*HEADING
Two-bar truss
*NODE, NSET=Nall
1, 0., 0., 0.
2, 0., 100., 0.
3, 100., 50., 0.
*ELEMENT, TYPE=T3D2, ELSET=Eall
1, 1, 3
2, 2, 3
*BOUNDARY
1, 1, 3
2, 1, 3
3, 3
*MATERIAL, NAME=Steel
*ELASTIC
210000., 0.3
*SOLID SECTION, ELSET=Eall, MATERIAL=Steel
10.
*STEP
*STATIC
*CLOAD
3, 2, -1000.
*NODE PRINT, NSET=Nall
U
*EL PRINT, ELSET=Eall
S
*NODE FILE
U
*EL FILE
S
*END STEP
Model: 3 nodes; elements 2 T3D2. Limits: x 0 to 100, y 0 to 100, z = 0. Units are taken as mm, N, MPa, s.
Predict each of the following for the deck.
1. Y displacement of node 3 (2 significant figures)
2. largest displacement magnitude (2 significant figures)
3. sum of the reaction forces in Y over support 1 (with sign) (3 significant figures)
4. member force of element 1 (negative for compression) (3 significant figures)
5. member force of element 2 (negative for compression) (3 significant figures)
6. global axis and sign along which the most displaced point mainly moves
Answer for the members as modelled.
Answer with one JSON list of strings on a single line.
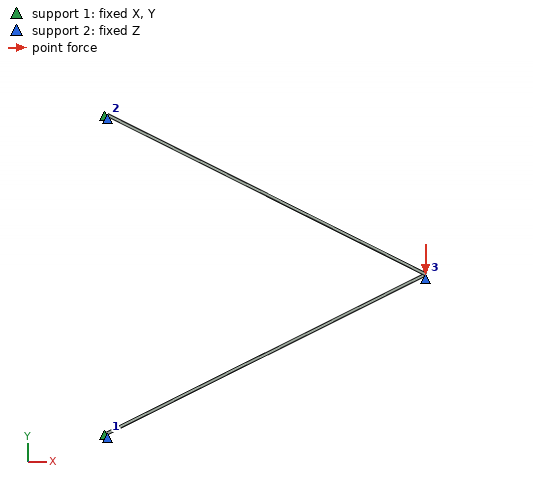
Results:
["-0.13 mm", "0.13 mm", "1000 N", "-1120 N", "1120 N", "-Y"]
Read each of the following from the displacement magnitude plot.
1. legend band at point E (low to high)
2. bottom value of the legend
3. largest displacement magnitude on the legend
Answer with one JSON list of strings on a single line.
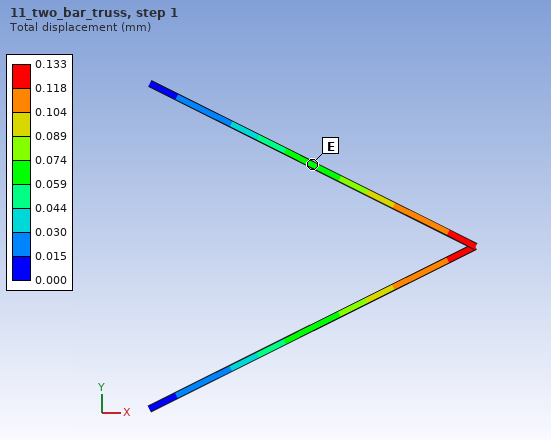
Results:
["0.059 to 0.074 mm", "0.000 mm", "0.133 mm"]
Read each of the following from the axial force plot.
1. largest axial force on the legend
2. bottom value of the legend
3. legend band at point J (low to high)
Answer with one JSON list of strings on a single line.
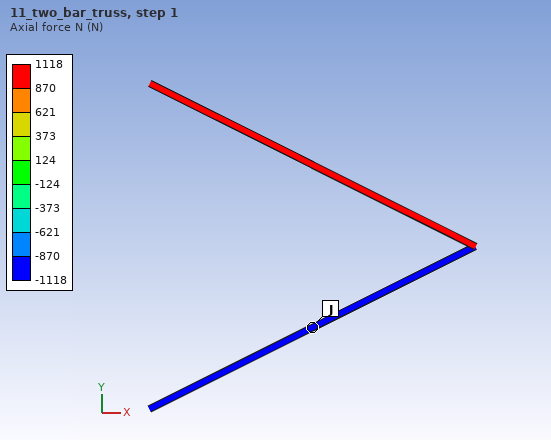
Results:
["1118 N", "-1118 N", "-1118 to -870 N"]
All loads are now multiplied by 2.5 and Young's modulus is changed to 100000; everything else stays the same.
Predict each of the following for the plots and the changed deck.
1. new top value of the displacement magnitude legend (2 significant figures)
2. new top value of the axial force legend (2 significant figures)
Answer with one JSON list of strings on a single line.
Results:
["0.70 mm", "2800 N"]
